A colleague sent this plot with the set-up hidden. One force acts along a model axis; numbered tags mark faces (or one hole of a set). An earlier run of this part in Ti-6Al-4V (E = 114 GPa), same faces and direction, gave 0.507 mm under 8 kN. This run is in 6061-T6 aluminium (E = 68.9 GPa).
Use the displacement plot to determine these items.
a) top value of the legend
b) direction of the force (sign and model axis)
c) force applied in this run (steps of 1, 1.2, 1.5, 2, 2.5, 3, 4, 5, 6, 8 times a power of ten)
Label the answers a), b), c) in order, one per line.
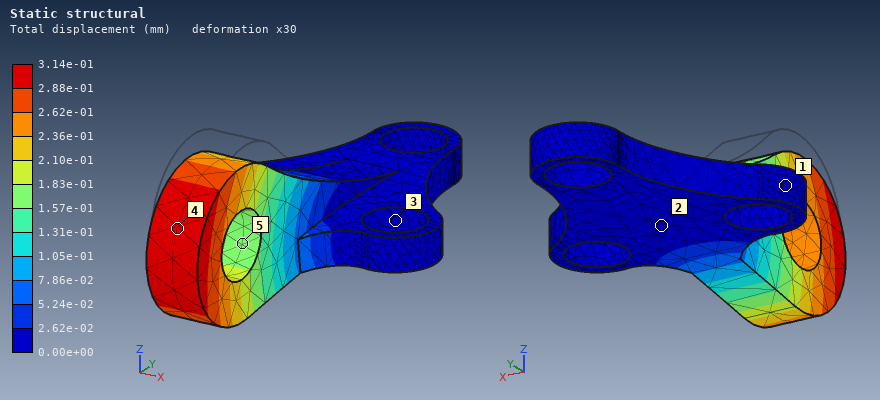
a) 3.14e-01 mm
b) -Z
c) 3 kN
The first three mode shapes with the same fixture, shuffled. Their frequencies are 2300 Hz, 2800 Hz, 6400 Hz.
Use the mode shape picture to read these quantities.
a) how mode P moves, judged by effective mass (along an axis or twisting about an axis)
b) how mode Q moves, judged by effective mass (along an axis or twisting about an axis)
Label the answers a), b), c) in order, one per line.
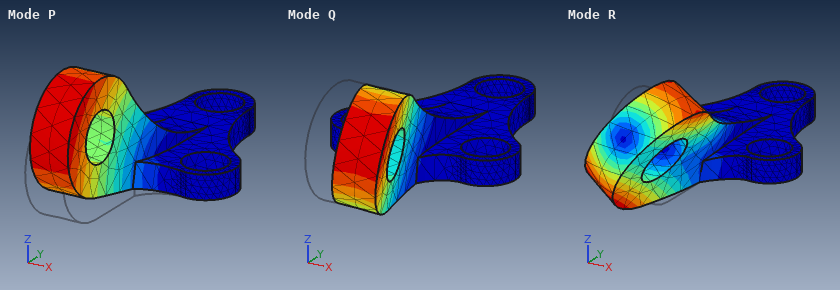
a) along Z
b) along X
